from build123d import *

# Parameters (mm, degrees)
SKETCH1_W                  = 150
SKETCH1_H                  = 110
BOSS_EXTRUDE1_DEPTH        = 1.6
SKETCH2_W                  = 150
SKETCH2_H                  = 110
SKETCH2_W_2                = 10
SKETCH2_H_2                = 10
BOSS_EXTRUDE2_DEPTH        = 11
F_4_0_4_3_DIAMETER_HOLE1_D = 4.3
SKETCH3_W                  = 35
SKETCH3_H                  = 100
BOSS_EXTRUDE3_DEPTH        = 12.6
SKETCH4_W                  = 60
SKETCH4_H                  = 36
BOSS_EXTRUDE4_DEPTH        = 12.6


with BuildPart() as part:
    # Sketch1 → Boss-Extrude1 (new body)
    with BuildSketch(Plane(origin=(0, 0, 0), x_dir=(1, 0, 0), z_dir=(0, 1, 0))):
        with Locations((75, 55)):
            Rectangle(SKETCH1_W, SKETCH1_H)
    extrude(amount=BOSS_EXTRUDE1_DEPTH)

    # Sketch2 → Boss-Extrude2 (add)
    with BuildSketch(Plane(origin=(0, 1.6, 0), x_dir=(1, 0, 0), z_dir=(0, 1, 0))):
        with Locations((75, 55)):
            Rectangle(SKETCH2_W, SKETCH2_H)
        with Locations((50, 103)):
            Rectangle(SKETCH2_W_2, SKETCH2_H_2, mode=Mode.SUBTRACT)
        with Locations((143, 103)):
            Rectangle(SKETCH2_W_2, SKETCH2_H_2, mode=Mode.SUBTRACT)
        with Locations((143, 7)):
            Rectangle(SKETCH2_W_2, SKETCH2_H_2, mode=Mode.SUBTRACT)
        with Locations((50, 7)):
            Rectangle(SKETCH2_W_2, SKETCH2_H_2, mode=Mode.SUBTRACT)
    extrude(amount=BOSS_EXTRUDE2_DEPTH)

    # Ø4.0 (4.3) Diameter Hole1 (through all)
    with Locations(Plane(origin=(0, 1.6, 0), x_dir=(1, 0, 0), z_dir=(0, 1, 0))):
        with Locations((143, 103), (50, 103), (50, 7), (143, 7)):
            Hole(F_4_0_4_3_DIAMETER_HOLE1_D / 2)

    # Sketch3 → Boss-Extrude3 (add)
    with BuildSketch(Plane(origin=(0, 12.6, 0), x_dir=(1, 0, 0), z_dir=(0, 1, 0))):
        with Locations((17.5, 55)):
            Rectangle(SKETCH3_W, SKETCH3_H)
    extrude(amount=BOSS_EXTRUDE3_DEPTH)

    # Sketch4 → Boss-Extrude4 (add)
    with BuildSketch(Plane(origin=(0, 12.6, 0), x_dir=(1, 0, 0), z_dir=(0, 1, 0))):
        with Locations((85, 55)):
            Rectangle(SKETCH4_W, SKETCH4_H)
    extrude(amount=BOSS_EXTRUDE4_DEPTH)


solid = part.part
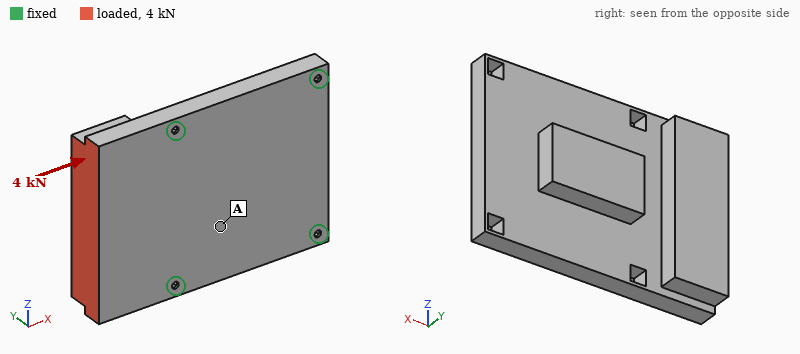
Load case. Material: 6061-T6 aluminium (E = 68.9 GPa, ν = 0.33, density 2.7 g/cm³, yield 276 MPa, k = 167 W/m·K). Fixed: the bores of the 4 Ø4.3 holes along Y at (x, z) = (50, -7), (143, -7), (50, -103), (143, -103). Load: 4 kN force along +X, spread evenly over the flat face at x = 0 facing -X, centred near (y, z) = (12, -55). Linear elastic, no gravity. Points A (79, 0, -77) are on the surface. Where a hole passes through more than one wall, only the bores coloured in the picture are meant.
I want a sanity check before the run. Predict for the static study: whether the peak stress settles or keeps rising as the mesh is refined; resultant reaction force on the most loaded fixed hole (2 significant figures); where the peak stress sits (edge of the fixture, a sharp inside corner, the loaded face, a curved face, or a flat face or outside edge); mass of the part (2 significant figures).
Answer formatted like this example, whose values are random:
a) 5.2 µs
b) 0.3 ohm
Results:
a) keeps rising
b) 1.1 kN
c) edge of the fixture
d) 740 g
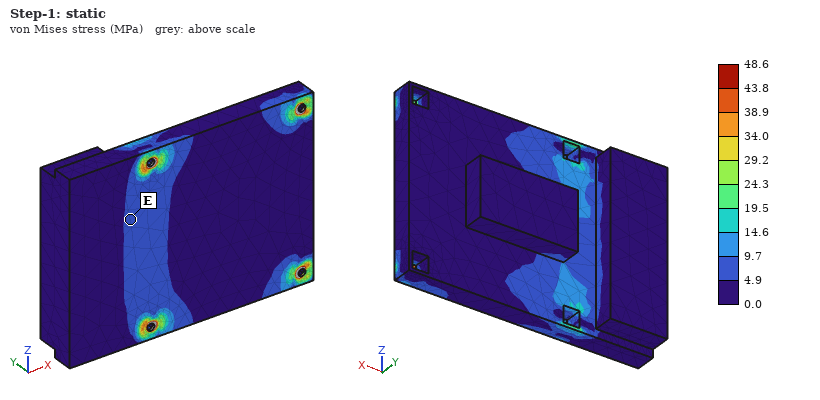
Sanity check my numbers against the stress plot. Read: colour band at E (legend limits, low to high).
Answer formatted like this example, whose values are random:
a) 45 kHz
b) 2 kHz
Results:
a) 4.9 to 9.7 MPa
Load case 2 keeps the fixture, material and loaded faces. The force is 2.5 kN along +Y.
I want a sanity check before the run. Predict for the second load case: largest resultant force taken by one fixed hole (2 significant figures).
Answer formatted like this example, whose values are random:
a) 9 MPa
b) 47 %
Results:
a) 2.6 kN
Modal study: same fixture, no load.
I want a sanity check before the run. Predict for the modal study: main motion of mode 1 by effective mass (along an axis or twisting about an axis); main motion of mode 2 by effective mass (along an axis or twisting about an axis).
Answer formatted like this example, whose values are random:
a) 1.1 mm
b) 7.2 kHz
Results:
a) along Y
b) along Y
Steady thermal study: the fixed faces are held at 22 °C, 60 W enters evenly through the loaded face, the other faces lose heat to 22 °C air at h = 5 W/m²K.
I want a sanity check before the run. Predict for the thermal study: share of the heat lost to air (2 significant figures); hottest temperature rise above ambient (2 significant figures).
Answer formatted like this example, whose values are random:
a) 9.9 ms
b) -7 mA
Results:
a) 5.6 %
b) 26 K
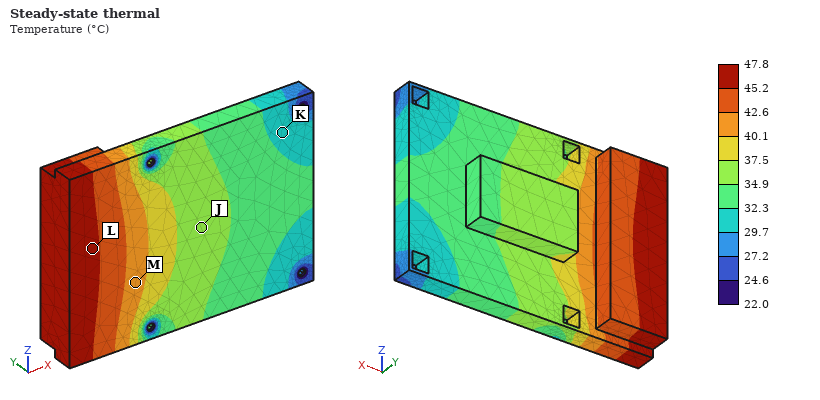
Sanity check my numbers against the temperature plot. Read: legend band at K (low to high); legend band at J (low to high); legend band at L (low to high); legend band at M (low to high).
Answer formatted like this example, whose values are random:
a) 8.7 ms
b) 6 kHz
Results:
a) 29.7 to 32.3 °C
b) 34.9 to 37.5 °C
c) 45.2 to 47.8 °C
d) 40.1 to 42.6 °C
